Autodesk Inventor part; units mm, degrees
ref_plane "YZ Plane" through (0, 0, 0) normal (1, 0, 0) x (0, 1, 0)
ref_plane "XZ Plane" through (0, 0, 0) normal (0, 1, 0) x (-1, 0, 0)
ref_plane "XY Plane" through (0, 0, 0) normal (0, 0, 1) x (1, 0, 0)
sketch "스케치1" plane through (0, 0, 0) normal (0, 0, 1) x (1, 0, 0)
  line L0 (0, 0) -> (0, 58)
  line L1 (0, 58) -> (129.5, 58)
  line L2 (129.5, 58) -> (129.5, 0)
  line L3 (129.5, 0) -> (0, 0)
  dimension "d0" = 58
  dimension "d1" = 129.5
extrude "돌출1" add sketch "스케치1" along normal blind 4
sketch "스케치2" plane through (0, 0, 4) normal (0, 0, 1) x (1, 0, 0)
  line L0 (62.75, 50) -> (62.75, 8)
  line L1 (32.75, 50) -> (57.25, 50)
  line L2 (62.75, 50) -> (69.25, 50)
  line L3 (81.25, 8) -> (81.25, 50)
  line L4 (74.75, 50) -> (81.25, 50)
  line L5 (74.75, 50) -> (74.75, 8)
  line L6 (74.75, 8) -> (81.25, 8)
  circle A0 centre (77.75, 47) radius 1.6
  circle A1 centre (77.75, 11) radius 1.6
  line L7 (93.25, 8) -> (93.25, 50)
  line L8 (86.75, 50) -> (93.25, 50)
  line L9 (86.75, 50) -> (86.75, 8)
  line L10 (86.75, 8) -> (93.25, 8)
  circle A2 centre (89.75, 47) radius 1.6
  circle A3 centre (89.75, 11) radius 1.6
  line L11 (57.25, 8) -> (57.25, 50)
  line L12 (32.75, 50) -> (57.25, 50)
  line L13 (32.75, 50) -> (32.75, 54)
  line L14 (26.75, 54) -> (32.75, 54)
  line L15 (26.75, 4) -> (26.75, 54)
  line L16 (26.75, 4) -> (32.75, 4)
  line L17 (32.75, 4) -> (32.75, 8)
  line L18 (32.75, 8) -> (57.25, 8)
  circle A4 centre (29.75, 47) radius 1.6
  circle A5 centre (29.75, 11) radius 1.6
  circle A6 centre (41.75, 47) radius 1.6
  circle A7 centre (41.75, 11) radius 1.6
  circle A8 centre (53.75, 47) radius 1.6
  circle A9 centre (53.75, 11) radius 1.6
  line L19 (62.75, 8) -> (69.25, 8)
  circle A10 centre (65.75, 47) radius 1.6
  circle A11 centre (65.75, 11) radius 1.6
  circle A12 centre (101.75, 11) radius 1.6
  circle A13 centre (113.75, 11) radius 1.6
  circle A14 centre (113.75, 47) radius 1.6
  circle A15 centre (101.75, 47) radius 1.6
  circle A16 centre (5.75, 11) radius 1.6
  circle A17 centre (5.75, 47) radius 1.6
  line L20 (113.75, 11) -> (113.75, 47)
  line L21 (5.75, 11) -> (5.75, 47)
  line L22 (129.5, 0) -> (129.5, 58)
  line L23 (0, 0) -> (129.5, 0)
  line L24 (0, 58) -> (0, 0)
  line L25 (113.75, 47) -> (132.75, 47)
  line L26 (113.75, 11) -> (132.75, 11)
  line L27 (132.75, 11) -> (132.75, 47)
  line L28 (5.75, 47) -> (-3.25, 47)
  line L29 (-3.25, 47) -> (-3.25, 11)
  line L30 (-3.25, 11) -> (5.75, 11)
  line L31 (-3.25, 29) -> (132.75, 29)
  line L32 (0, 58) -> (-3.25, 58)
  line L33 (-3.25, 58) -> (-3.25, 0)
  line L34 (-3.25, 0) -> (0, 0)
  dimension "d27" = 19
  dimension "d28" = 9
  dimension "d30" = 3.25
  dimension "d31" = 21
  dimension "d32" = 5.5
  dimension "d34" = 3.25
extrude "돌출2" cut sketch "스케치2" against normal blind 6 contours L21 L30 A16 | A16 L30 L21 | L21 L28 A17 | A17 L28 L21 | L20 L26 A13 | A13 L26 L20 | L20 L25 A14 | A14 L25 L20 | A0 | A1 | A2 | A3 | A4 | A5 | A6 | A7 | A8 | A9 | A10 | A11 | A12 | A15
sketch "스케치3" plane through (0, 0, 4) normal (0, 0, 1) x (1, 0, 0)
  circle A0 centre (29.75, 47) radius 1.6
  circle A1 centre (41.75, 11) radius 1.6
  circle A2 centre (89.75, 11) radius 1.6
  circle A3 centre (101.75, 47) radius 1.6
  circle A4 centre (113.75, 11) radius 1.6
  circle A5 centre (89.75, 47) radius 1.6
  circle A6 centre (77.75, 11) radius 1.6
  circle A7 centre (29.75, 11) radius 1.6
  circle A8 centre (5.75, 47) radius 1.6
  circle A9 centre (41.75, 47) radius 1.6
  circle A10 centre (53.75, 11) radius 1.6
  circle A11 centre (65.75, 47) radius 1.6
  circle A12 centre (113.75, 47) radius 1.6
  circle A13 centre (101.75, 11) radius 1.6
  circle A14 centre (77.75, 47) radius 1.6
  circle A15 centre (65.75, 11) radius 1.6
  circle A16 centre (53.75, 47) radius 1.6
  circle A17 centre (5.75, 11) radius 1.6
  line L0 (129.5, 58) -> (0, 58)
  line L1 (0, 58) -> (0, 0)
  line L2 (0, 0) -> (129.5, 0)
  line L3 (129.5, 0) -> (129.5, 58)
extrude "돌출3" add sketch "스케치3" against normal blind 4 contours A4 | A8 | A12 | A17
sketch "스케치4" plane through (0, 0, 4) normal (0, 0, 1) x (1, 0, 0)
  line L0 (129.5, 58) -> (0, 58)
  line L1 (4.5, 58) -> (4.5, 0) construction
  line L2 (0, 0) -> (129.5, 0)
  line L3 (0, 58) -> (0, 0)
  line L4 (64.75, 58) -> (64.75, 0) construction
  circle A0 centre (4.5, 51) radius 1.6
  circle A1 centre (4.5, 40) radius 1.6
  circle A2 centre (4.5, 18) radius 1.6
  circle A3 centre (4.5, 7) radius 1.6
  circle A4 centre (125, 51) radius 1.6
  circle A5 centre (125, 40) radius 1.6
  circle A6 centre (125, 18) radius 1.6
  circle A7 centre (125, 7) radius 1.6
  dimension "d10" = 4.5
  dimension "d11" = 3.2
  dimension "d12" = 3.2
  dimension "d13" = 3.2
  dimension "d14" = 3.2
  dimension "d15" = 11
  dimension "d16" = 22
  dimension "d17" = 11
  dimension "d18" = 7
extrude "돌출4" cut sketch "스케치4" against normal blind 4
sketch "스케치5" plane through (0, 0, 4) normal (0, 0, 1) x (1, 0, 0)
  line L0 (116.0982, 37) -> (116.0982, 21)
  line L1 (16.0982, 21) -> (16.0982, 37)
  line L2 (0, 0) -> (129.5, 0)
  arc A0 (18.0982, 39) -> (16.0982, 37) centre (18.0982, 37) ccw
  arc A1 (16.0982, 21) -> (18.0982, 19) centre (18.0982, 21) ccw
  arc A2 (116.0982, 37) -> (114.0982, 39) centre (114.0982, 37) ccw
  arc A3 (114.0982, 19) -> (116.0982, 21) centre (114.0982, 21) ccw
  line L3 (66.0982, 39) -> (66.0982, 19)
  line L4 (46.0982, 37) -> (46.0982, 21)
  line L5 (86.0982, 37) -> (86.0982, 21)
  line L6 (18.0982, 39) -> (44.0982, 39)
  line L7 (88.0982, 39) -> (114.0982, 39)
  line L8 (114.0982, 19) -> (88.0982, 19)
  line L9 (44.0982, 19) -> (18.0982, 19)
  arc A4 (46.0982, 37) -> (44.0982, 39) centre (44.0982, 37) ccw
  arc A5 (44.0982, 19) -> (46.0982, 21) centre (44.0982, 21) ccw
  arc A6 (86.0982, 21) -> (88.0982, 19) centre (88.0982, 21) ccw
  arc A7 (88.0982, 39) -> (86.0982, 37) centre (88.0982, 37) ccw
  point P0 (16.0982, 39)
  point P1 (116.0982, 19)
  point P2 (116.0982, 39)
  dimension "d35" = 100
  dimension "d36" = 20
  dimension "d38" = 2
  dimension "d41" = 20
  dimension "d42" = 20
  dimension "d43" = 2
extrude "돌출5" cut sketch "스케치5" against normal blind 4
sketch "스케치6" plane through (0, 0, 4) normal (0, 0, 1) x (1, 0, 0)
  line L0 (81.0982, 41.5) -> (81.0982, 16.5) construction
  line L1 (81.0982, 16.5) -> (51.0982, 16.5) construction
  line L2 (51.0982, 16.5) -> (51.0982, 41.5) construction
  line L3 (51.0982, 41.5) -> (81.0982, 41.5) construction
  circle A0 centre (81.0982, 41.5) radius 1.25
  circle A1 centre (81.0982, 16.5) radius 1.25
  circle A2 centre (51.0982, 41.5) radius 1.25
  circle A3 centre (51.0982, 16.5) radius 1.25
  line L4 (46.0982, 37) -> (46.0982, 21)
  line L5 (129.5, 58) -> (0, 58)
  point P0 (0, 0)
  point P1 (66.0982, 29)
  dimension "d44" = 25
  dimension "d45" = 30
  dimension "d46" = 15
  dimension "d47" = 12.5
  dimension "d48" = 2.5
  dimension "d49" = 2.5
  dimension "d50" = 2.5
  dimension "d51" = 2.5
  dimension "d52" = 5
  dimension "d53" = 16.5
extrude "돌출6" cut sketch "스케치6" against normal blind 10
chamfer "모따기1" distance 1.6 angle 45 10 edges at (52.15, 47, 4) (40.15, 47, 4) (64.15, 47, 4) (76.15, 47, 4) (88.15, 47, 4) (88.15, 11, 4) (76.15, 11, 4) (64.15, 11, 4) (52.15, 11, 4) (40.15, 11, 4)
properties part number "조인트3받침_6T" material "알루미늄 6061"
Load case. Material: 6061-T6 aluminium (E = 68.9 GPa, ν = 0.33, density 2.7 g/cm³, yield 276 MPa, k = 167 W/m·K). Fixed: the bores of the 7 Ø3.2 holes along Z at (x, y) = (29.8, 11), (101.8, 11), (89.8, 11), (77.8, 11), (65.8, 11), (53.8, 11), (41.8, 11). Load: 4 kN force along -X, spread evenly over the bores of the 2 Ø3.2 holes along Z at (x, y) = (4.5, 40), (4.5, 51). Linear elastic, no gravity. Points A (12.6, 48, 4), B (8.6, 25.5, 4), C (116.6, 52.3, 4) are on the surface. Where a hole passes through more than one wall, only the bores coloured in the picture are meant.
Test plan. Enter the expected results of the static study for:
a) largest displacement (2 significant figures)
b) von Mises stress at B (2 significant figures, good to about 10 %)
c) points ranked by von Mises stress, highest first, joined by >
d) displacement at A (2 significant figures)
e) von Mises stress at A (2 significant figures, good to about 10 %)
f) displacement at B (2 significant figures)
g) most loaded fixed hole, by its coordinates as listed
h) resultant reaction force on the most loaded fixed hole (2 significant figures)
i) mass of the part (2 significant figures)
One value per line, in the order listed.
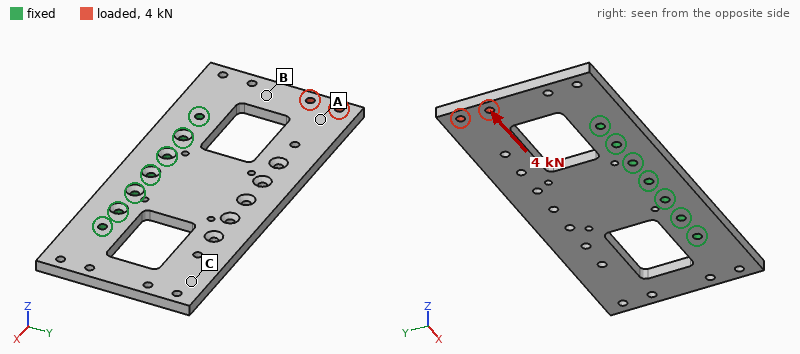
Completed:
0.11 mm
26 MPa
A > B > C
0.091 mm
57 MPa
0.059 mm
(29.8, 11)
1.4 kN
66 g
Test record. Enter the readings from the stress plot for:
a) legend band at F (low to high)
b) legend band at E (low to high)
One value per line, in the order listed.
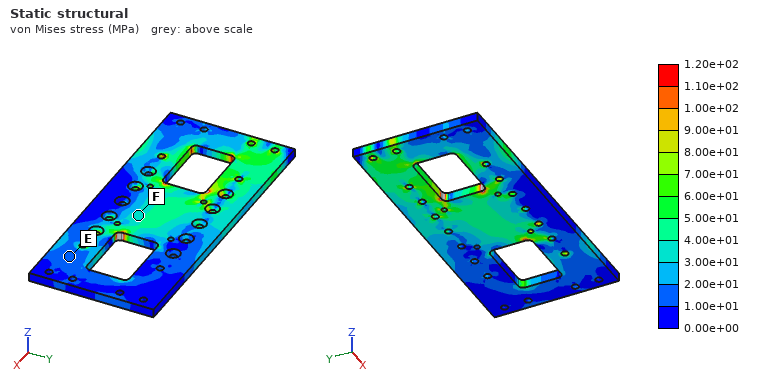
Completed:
3.00e+01 to 4.00e+01 MPa
1.00e+01 to 2.00e+01 MPa
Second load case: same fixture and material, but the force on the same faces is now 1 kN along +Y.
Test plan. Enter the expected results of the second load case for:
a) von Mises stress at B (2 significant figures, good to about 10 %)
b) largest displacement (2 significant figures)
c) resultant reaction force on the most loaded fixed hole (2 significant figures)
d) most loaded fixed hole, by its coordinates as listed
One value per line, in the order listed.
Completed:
20 MPa
41 µm
1.3 kN
(29.8, 11)
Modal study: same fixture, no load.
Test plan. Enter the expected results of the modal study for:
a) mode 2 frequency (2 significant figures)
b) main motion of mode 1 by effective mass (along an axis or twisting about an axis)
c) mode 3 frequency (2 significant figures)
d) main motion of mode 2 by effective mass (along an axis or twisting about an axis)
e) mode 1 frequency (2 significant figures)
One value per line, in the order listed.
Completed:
1200 Hz
along Z
2000 Hz
twisting about Y
980 Hz
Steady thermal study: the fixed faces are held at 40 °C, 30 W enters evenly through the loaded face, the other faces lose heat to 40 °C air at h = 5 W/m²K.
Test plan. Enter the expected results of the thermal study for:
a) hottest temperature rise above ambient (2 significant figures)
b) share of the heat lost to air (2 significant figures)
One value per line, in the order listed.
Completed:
80 K
4.0 %
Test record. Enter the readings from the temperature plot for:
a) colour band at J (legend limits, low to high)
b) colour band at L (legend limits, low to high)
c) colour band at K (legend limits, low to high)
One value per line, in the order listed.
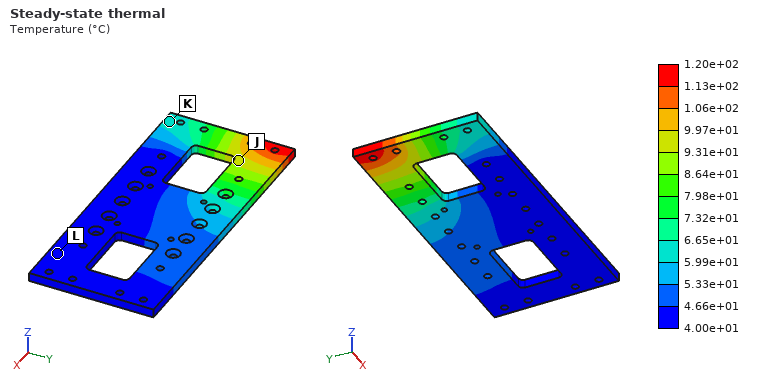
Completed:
9.31e+01 to 9.97e+01 °C
4.00e+01 to 4.66e+01 °C
5.99e+01 to 6.65e+01 °C
